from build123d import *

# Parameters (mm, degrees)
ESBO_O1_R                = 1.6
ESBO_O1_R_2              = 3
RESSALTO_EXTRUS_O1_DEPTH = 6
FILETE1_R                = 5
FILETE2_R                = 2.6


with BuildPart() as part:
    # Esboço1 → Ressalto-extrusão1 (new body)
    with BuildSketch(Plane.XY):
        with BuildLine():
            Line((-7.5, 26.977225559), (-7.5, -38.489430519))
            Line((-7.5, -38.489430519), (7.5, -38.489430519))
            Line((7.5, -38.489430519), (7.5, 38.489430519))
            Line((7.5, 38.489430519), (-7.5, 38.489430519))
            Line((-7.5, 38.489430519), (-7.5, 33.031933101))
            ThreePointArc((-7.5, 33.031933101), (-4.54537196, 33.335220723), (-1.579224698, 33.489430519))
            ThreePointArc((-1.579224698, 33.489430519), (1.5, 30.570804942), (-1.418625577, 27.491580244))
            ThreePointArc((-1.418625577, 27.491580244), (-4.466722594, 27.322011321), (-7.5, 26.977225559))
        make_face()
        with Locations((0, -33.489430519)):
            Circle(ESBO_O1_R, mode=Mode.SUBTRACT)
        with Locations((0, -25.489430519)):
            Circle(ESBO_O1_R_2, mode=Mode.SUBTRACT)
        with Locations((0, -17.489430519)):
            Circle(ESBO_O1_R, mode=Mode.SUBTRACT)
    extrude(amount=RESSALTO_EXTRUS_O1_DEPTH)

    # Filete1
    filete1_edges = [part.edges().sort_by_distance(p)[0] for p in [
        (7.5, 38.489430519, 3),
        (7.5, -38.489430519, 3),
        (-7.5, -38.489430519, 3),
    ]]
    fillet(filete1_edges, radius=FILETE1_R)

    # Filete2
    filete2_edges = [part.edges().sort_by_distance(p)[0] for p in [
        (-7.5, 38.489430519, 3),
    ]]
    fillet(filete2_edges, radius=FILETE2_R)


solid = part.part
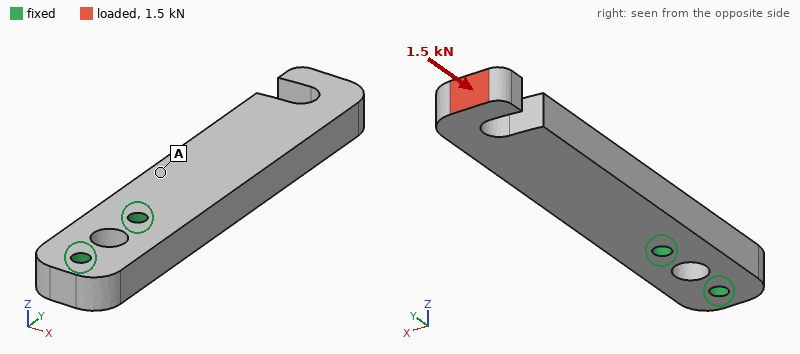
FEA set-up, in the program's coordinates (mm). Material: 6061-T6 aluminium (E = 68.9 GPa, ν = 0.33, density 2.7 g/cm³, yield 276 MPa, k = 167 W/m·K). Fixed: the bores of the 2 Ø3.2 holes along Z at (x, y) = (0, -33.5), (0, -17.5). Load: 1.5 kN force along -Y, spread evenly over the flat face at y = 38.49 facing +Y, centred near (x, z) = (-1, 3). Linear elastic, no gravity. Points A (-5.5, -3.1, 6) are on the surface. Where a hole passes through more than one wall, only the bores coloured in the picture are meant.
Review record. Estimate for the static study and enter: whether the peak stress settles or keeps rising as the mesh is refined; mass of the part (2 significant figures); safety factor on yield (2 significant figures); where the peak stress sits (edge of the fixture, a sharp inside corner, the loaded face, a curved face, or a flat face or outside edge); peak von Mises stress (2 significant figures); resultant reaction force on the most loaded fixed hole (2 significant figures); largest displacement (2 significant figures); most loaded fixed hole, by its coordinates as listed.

settles
17 g
0.68
a curved face
410 MPa
1.3 kN
0.18 mm
(0, -17.5)
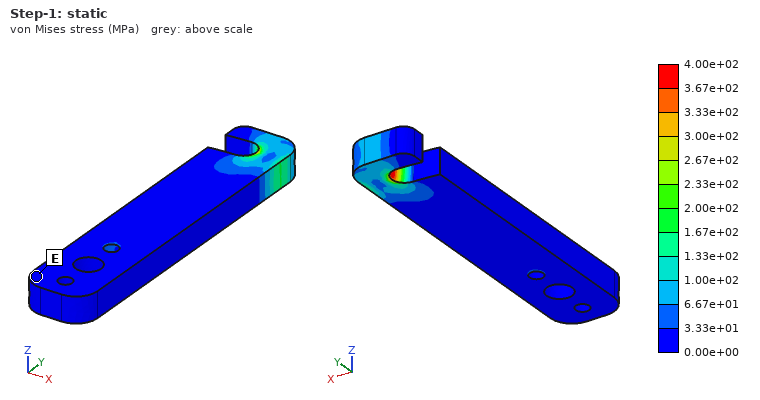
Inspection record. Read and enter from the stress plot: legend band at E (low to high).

0.00e+00 to 3.33e+01 MPa
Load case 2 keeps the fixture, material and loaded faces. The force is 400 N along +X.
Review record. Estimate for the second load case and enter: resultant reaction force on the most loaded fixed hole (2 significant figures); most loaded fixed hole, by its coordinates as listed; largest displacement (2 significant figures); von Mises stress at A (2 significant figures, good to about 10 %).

1.2 kN
(0, -17.5)
0.34 mm
54 MPa
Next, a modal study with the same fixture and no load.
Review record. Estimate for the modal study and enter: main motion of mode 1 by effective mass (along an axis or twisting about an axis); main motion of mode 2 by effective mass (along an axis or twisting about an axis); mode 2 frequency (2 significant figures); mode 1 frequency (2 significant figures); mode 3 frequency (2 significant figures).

along Z
along X
3300 Hz
1700 Hz
8900 Hz
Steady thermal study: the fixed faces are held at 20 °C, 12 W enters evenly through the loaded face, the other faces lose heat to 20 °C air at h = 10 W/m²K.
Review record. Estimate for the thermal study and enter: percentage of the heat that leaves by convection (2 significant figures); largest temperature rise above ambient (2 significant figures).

4.8 %
63 K
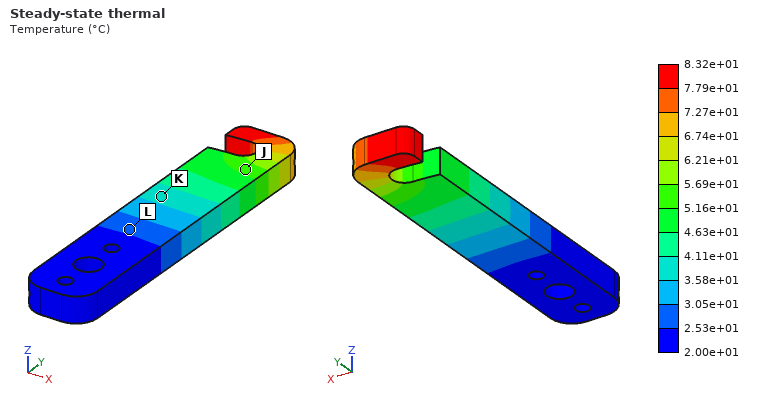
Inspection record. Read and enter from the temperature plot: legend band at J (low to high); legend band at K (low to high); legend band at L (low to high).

5.16e+01 to 5.69e+01 °C
3.58e+01 to 4.11e+01 °C
2.53e+01 to 3.05e+01 °C
